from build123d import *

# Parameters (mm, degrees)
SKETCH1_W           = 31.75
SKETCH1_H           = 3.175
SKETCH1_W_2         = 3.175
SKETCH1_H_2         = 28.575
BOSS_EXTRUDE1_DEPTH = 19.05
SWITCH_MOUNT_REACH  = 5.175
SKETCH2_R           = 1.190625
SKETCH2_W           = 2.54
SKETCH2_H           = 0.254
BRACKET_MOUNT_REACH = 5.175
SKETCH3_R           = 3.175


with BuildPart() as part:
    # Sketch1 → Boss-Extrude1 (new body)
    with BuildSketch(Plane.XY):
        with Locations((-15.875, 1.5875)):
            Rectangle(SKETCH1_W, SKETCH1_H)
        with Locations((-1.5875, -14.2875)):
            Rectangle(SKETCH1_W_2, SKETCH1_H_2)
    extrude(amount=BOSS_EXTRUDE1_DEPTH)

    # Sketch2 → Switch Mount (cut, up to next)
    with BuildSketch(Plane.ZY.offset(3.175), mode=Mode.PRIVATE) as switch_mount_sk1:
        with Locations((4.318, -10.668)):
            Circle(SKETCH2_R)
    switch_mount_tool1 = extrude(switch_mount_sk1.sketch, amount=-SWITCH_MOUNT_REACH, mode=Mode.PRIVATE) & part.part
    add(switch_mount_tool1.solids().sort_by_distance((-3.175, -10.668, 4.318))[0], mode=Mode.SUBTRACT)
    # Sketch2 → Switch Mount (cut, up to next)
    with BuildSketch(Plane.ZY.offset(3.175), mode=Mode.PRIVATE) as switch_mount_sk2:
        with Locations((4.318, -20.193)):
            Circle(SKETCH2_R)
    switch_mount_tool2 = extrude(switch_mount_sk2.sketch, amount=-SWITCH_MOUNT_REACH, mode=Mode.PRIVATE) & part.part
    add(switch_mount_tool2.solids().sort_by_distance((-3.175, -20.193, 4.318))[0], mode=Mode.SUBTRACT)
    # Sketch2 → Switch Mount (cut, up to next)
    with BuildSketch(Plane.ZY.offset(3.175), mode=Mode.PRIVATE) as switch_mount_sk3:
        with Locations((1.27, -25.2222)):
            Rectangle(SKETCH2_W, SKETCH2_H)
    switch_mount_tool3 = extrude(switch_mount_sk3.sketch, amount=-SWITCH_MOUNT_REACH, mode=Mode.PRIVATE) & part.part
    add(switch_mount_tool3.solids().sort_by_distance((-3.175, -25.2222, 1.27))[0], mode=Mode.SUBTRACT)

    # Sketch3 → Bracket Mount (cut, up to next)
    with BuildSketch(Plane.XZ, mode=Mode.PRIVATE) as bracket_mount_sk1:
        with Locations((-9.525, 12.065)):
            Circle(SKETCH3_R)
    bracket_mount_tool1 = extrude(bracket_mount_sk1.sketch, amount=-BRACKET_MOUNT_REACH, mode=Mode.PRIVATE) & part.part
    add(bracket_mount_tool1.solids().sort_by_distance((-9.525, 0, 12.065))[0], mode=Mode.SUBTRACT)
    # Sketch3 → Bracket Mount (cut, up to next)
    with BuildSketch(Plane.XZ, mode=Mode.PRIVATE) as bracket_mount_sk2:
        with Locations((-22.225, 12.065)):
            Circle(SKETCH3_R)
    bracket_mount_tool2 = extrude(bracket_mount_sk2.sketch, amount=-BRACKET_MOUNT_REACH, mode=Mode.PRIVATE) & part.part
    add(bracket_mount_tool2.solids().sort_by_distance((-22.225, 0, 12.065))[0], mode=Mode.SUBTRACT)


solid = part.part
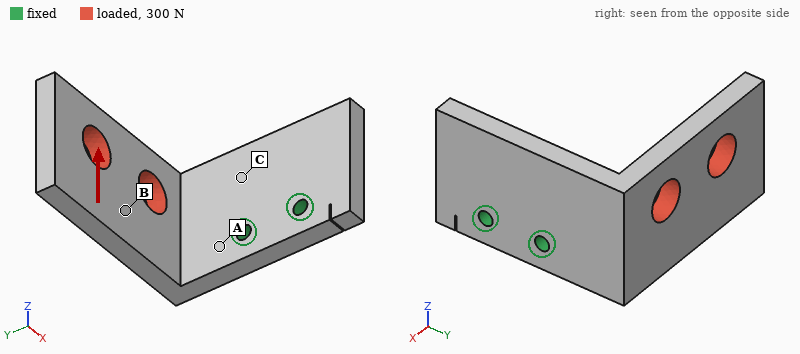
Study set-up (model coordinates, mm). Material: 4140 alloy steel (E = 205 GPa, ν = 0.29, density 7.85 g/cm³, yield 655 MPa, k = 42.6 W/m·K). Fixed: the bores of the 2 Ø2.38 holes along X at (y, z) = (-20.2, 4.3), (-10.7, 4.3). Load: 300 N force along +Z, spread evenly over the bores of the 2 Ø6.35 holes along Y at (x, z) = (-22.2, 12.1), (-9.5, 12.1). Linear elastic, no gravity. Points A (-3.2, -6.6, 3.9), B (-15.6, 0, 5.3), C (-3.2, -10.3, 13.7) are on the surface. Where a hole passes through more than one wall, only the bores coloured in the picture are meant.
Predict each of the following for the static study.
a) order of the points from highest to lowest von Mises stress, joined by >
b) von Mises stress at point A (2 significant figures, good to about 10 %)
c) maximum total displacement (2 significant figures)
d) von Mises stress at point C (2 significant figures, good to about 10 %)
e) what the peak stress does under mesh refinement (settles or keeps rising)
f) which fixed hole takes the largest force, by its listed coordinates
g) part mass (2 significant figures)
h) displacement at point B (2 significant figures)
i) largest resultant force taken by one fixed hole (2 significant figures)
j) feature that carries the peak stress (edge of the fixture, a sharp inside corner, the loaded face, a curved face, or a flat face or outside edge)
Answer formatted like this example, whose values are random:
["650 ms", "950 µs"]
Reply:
["A > C > B", "140 MPa", "0.13 mm", "63 MPa", "keeps rising", "(-10.7, 4.3)", "27 g", "0.057 mm", "590 N", "edge of the fixture"]
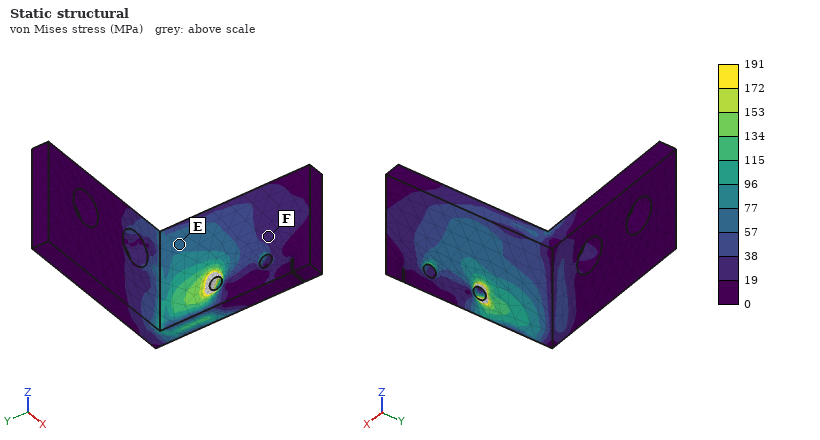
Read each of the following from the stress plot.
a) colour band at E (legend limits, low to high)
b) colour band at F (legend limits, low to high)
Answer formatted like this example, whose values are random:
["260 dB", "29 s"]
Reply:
["57 to 77 MPa", "19 to 38 MPa"]
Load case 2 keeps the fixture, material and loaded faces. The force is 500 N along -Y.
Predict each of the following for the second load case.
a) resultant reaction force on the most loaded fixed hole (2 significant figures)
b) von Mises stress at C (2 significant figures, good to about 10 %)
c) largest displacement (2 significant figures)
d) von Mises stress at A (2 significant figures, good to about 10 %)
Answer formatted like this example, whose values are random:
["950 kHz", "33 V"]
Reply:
["550 N", "160 MPa", "0.45 mm", "260 MPa"]
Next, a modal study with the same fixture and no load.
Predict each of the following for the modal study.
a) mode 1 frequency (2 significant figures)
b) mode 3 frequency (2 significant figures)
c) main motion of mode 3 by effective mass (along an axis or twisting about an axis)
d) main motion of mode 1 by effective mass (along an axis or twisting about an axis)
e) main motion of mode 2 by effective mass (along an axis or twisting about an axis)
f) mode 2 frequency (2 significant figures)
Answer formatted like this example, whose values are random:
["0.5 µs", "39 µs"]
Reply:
["1700 Hz", "6200 Hz", "along X", "along Y", "along Z", "2500 Hz"]
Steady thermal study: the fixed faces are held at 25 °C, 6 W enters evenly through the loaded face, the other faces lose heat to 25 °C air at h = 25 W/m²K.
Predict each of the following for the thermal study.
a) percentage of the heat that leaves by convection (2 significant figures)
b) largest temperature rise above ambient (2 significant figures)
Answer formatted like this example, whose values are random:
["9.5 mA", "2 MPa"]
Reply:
["29 %", "57 K"]
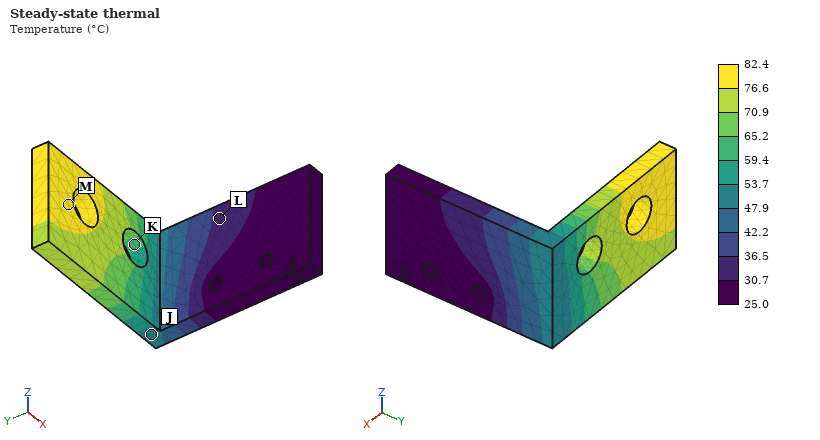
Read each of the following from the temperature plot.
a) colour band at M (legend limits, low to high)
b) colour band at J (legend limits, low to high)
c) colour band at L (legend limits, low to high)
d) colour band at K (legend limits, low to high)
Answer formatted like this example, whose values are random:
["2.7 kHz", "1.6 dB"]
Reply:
["76.6 to 82.4 °C", "47.9 to 53.7 °C", "30.7 to 36.5 °C", "59.4 to 65.2 °C"]
